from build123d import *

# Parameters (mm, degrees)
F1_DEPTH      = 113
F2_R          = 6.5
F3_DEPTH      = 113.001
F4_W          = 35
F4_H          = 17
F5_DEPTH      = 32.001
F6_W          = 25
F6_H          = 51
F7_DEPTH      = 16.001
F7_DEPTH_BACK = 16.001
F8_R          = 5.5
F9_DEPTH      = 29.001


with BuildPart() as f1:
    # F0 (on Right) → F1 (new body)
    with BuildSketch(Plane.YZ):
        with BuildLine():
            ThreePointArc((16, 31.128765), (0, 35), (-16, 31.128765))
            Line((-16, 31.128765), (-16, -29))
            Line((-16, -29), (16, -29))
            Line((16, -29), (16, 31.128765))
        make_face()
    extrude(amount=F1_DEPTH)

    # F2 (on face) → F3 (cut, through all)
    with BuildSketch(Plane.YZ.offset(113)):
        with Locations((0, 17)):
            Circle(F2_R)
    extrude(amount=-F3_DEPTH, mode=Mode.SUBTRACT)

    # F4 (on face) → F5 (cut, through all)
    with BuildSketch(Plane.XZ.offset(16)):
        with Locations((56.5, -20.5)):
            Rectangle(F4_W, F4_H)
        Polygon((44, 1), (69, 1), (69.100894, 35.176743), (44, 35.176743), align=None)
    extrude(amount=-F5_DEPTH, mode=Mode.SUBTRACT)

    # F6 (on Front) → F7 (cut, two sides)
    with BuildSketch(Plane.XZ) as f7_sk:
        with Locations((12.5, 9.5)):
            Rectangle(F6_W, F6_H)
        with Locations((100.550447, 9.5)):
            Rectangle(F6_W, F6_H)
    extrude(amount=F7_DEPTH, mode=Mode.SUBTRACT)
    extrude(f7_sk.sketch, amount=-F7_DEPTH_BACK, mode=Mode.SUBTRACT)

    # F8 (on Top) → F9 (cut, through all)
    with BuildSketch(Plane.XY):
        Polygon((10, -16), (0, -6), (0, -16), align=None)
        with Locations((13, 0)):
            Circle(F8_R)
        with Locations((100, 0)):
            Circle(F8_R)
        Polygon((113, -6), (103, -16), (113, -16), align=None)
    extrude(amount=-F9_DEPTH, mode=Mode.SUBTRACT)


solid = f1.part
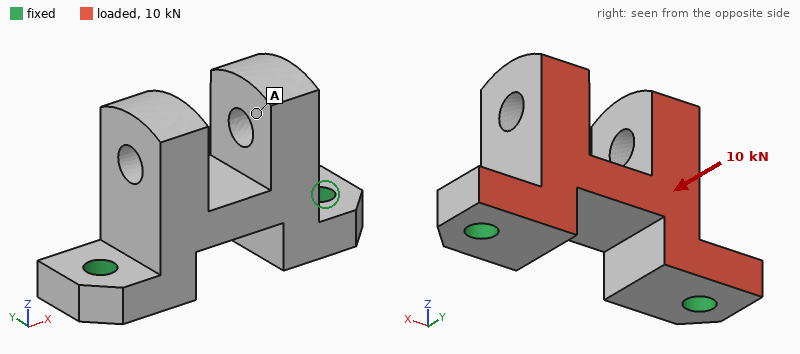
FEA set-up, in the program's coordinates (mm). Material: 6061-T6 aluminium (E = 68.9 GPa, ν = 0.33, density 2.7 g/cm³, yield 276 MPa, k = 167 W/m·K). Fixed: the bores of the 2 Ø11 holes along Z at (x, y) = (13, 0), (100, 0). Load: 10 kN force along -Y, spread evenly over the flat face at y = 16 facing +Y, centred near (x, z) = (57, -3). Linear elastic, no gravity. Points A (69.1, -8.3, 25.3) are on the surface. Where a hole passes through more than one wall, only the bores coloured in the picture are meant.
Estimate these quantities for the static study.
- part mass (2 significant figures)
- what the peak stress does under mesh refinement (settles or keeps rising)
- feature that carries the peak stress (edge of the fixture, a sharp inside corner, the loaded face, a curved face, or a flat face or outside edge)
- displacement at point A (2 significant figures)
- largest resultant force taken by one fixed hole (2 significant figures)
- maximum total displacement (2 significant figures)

250 g
keeps rising
edge of the fixture
0.15 mm
5.0 kN
0.18 mm
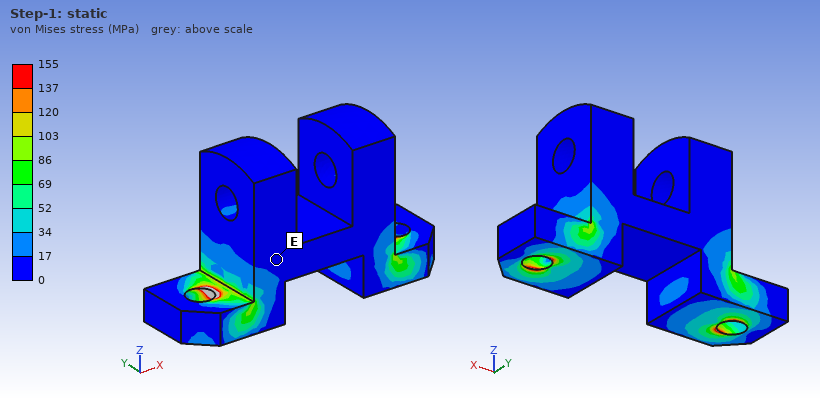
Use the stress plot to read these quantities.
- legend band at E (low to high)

0 to 17 MPa
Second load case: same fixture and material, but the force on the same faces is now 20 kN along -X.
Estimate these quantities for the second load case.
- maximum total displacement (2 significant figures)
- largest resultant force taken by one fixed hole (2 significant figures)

0.13 mm
12 kN
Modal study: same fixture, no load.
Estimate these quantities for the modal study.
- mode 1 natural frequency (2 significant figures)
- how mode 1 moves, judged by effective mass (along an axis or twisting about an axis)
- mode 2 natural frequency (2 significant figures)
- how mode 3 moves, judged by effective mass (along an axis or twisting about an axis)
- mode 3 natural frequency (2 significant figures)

2800 Hz
along Y
4700 Hz
along X
5700 Hz
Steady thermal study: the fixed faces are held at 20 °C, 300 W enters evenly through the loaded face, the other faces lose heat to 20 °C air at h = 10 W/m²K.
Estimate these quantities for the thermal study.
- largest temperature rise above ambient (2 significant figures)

62 K
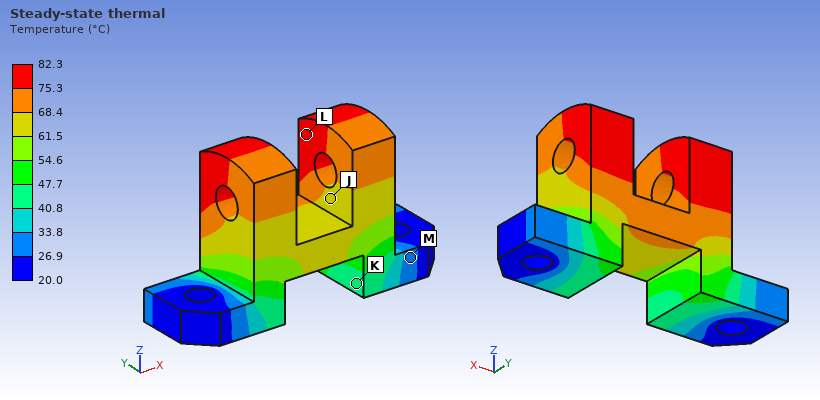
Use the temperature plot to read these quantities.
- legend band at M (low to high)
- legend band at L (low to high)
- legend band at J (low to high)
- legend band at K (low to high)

26.9 to 33.8 °C
75.3 to 82.3 °C
61.5 to 68.4 °C
40.8 to 47.7 °C
